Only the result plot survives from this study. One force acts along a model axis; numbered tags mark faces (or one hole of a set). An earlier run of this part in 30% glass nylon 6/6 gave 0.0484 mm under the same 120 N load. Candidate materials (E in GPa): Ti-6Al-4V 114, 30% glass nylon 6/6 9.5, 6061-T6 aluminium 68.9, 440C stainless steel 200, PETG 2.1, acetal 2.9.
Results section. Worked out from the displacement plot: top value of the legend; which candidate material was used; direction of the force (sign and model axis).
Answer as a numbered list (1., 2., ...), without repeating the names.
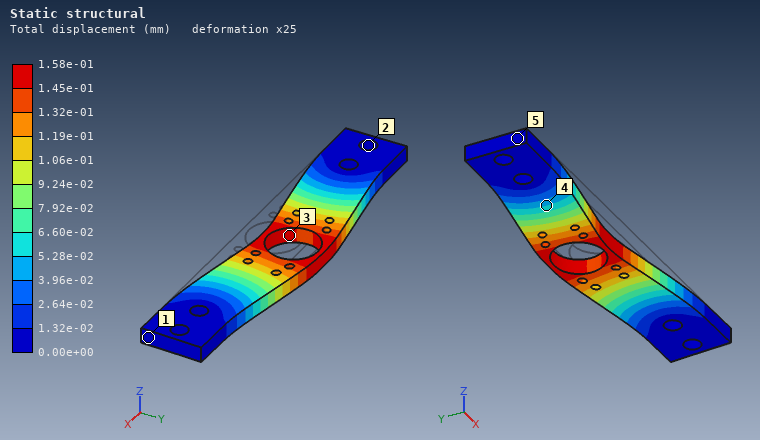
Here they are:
1. 1.58e-01 mm
2. acetal
3. +Y
